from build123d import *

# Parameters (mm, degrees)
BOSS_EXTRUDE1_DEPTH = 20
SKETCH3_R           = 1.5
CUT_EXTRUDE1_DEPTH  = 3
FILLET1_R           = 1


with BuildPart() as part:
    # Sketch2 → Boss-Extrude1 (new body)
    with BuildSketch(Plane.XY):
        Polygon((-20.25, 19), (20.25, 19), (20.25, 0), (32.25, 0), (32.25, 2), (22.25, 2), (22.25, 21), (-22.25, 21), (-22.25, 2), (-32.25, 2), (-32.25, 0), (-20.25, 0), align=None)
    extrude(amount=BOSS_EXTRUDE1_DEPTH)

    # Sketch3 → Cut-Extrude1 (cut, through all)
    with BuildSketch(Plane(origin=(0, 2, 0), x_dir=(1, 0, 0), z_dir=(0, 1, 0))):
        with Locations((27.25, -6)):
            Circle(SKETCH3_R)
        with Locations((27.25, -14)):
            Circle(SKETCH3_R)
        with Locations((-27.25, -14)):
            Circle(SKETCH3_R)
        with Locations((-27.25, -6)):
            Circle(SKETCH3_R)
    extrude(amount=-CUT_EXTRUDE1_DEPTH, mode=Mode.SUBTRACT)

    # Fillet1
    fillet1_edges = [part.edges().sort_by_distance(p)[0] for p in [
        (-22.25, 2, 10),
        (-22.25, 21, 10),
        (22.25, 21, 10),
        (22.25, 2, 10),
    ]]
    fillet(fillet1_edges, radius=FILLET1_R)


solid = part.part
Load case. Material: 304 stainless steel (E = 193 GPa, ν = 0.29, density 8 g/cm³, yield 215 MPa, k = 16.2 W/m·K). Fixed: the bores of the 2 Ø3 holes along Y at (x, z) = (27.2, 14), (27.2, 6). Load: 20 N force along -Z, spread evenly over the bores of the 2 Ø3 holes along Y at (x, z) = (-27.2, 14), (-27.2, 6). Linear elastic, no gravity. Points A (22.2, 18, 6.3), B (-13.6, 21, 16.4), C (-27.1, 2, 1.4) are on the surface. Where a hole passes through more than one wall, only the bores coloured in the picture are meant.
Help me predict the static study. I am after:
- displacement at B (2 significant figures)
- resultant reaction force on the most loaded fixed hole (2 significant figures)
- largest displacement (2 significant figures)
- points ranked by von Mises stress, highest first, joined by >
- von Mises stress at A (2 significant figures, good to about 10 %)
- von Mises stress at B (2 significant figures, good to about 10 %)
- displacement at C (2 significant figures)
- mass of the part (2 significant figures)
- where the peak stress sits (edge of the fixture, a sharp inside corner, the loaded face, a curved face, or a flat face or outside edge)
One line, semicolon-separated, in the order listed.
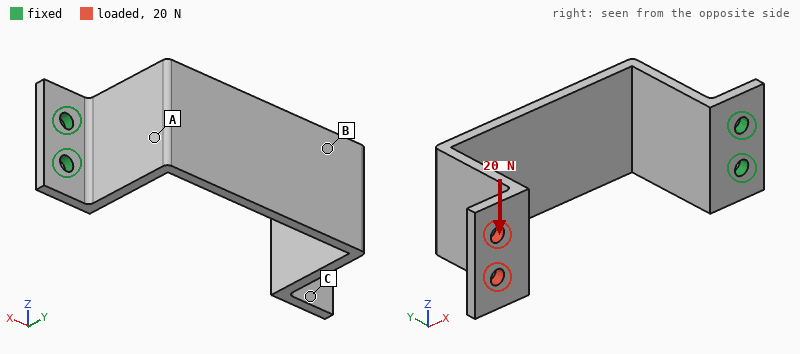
0.13 mm; 100 N; 0.30 mm; A > B > C; 52 MPa; 21 MPa; 0.27 mm; 32 g; a curved face
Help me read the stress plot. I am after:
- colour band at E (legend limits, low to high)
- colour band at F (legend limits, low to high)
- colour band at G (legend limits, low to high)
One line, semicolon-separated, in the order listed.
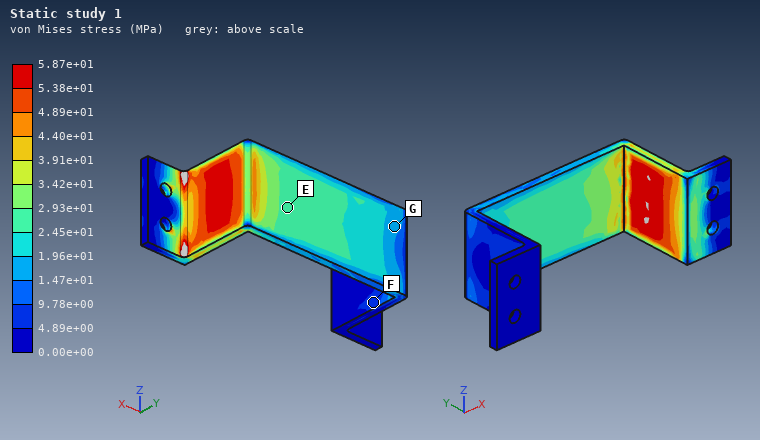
2.45e+01 to 2.93e+01 MPa; 4.89e+00 to 9.78e+00 MPa; 1.47e+01 to 1.96e+01 MPa
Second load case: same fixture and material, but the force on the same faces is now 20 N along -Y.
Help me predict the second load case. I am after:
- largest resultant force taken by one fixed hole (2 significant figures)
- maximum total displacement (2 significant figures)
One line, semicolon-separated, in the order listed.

16 N; 0.82 mm
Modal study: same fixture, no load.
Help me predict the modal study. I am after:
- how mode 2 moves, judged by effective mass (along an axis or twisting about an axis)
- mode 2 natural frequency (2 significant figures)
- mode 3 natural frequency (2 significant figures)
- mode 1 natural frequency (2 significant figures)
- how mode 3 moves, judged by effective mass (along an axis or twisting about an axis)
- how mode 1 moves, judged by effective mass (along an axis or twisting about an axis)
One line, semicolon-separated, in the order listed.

along Z; 470 Hz; 870 Hz; 250 Hz; along X; along Y
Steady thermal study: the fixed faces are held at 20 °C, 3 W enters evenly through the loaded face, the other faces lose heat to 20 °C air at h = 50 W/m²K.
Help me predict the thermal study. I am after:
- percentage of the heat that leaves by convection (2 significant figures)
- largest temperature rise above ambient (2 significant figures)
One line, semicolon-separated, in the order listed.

99 %; 66 K
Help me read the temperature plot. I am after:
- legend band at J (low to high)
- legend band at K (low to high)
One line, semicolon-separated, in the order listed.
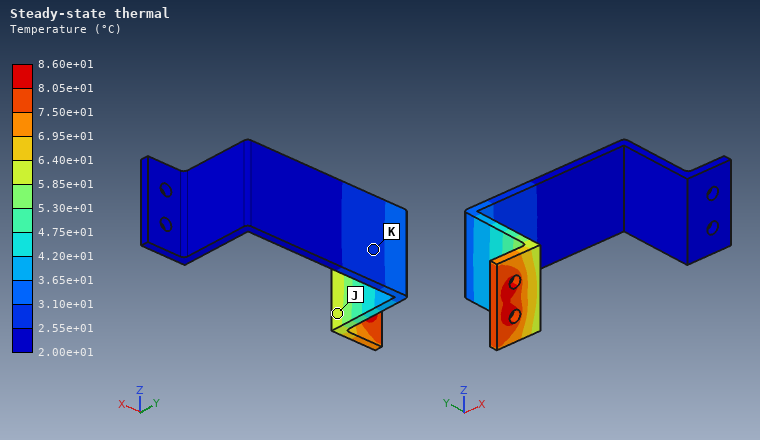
5.85e+01 to 6.40e+01 °C; 2.55e+01 to 3.10e+01 °C
